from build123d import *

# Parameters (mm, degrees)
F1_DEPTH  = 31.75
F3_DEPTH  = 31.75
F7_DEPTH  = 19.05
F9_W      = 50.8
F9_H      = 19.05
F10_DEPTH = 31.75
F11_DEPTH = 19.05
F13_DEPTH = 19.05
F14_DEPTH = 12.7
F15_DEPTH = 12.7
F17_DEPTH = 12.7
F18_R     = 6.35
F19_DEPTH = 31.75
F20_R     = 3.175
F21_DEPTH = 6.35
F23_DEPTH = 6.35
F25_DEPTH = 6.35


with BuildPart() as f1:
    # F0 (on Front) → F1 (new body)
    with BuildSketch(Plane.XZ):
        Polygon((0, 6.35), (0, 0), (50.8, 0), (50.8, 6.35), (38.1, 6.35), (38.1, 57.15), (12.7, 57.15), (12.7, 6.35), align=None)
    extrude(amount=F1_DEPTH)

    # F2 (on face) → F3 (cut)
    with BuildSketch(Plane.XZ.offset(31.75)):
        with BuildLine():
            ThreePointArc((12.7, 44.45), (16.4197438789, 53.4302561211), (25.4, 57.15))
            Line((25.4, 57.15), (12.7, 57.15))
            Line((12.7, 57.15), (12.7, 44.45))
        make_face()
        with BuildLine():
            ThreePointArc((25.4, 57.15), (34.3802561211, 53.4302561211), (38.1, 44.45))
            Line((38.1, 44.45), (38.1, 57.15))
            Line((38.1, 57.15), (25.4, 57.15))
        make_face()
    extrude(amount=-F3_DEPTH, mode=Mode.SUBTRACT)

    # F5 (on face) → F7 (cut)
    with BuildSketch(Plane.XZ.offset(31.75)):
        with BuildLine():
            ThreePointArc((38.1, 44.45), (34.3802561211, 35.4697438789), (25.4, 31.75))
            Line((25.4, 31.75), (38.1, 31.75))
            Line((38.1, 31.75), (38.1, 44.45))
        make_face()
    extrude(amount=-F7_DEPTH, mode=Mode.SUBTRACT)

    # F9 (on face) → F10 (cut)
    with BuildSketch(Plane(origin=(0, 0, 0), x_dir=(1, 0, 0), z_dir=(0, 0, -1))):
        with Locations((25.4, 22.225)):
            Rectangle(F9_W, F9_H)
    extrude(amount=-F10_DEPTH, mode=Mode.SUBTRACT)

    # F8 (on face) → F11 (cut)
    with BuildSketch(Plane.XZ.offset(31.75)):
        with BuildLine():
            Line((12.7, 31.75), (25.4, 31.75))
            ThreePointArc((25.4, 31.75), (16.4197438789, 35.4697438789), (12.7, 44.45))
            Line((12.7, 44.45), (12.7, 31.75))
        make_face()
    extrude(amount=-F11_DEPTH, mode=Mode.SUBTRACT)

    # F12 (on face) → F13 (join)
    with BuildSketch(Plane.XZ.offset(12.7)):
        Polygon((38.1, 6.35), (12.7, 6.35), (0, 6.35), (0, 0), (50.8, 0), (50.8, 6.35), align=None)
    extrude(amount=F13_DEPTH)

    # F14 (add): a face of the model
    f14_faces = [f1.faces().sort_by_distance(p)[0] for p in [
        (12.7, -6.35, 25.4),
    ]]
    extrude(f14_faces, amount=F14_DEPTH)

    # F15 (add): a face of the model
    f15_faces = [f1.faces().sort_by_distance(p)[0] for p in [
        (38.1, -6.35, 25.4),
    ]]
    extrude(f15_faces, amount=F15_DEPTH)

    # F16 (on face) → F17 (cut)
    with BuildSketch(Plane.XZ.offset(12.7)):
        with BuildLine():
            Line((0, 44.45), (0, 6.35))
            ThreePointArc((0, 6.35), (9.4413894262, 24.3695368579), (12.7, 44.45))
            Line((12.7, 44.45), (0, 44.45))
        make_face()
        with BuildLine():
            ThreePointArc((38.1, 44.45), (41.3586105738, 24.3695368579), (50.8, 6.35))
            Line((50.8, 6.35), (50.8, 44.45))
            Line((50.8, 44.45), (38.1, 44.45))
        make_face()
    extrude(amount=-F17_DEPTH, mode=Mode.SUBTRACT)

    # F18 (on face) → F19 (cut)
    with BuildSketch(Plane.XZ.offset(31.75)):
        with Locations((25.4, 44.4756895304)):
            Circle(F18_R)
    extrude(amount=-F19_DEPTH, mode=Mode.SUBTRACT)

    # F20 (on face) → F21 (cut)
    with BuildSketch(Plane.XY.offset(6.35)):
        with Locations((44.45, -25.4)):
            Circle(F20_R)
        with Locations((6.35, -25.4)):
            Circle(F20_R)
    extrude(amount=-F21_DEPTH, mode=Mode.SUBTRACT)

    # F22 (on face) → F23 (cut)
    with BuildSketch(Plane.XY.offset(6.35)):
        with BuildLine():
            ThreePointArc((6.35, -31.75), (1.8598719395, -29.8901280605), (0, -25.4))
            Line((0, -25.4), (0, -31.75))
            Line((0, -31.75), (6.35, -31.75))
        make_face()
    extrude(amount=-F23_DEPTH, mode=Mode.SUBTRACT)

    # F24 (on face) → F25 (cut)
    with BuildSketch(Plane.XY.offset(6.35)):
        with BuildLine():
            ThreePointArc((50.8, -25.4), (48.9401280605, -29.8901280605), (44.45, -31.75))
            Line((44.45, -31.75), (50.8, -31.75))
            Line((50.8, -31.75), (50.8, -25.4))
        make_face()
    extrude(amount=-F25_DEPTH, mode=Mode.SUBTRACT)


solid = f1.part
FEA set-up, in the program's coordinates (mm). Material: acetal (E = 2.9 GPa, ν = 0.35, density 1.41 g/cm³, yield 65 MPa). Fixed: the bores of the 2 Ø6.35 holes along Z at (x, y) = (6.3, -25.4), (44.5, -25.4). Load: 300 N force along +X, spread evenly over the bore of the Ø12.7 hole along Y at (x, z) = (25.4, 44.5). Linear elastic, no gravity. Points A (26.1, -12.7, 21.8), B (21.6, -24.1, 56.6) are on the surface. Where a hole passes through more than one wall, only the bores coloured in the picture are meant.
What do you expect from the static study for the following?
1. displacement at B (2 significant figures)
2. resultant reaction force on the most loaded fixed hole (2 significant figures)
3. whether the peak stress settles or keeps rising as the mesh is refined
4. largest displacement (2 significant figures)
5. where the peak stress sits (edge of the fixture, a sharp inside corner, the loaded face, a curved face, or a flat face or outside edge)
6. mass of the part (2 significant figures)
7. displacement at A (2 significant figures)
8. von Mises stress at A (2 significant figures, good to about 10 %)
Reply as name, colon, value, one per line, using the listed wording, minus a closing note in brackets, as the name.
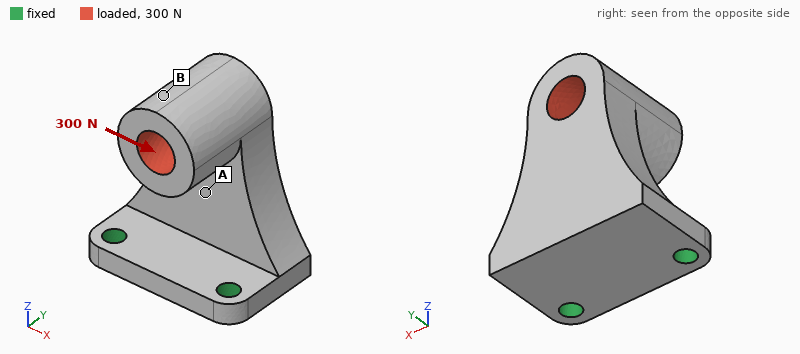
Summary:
displacement at B: 0.68 mm
resultant reaction force on the most loaded fixed hole: 360 N
whether the peak stress settles or keeps rising as the mesh is refined: keeps rising
largest displacement: 0.75 mm
where the peak stress sits: edge of the fixture
mass of the part: 49 g
displacement at A: 0.20 mm
von Mises stress at A: 5.5 MPa
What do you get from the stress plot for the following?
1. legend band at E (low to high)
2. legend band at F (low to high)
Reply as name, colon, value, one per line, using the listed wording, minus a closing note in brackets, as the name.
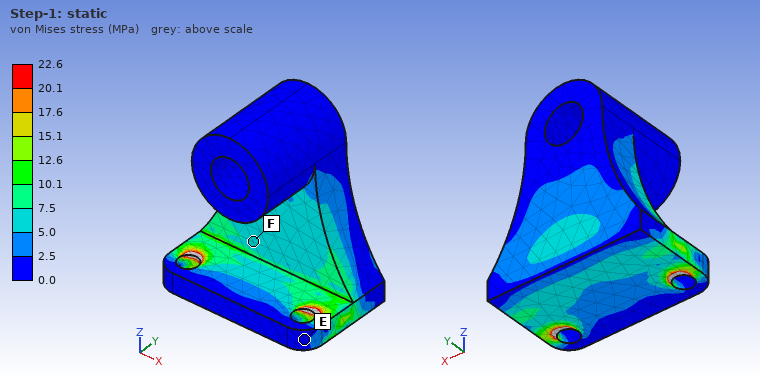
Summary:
legend band at E: 0.0 to 2.5 MPa
legend band at F: 5.0 to 7.5 MPa
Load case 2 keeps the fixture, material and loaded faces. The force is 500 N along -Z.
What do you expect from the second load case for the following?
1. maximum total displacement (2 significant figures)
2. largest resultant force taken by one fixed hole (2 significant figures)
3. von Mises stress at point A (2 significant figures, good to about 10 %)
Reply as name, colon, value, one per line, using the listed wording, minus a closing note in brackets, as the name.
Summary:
maximum total displacement: 0.32 mm
largest resultant force taken by one fixed hole: 250 N
von Mises stress at point A: 5.9 MPa
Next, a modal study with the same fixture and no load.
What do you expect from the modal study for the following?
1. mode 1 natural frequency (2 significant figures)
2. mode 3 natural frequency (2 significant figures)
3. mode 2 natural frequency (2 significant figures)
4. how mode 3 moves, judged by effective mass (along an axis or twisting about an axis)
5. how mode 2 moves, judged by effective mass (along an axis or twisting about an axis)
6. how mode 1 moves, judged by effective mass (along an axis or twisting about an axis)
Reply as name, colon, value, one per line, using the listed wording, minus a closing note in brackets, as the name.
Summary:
mode 1 natural frequency: 340 Hz
mode 3 natural frequency: 1400 Hz
mode 2 natural frequency: 840 Hz
how mode 3 moves, judged by effective mass: along Z
how mode 2 moves, judged by effective mass: along X
how mode 1 moves, judged by effective mass: along Y
